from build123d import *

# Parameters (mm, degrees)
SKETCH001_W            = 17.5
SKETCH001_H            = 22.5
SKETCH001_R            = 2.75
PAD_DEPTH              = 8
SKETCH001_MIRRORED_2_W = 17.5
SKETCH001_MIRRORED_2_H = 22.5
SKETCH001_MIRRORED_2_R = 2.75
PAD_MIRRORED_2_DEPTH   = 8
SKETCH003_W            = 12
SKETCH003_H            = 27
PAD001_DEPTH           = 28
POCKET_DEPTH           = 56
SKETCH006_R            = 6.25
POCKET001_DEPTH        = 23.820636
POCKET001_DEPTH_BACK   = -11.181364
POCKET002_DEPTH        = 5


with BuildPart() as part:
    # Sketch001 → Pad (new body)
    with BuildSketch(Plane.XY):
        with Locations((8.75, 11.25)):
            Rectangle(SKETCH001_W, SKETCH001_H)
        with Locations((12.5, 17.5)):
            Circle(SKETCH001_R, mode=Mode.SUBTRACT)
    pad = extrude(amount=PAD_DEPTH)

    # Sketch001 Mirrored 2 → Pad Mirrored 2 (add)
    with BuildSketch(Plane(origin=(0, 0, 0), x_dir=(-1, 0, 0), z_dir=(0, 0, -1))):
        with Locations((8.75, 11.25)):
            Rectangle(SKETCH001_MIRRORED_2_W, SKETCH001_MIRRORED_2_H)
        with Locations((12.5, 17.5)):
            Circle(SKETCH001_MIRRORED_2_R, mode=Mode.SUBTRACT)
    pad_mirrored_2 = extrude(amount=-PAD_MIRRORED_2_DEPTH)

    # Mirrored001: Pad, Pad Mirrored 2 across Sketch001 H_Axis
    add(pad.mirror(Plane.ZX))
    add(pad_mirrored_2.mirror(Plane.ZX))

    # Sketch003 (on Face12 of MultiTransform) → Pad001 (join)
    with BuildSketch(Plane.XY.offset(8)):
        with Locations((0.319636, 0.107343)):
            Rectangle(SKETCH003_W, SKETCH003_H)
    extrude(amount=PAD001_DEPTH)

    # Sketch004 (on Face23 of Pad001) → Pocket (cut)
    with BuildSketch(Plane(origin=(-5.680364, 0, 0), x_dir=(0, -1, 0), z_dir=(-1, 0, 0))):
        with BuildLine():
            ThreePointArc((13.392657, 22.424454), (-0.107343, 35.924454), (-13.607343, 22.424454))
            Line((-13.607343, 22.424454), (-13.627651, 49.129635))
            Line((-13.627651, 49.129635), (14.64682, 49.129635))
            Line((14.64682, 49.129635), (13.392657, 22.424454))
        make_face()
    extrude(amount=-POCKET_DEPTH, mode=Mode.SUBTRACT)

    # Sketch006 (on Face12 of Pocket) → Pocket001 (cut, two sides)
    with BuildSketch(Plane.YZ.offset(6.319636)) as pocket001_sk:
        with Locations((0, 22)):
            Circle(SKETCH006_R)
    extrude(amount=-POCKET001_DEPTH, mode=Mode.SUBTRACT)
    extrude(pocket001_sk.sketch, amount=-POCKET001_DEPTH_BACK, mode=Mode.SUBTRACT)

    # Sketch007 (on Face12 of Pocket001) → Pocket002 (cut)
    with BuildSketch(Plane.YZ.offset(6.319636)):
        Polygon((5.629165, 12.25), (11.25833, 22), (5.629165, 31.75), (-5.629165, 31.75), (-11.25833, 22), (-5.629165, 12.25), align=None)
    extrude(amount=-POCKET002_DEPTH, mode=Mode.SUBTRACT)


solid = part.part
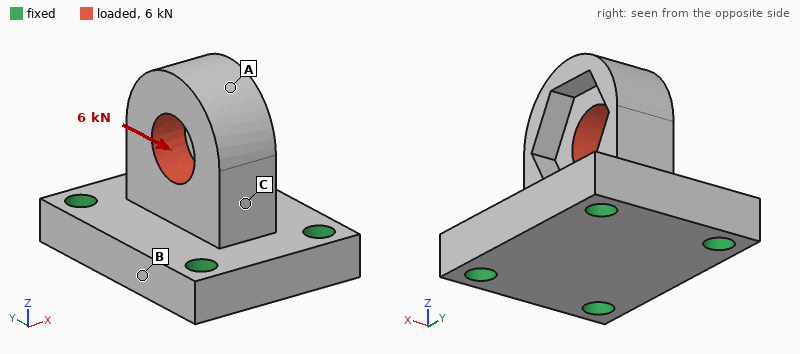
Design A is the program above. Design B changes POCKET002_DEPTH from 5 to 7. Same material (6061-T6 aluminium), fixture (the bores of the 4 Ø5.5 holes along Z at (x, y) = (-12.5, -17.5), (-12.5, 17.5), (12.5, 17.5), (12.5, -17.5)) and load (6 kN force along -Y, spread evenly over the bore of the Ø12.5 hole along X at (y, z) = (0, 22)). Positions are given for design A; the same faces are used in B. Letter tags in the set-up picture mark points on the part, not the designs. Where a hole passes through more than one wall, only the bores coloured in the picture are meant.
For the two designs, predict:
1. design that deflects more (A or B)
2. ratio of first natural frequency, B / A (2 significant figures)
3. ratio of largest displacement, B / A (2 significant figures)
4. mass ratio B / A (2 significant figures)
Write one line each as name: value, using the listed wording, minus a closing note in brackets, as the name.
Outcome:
design that deflects more: B
ratio of first natural frequency, B / A: 0.99
ratio of largest displacement, B / A: 1.2
mass ratio B / A: 0.98
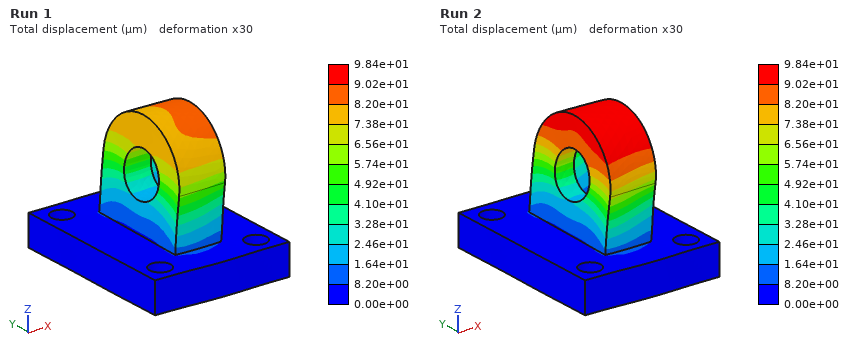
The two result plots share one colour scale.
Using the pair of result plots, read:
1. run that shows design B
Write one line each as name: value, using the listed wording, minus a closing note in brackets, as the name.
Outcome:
run that shows design B: Run 2
